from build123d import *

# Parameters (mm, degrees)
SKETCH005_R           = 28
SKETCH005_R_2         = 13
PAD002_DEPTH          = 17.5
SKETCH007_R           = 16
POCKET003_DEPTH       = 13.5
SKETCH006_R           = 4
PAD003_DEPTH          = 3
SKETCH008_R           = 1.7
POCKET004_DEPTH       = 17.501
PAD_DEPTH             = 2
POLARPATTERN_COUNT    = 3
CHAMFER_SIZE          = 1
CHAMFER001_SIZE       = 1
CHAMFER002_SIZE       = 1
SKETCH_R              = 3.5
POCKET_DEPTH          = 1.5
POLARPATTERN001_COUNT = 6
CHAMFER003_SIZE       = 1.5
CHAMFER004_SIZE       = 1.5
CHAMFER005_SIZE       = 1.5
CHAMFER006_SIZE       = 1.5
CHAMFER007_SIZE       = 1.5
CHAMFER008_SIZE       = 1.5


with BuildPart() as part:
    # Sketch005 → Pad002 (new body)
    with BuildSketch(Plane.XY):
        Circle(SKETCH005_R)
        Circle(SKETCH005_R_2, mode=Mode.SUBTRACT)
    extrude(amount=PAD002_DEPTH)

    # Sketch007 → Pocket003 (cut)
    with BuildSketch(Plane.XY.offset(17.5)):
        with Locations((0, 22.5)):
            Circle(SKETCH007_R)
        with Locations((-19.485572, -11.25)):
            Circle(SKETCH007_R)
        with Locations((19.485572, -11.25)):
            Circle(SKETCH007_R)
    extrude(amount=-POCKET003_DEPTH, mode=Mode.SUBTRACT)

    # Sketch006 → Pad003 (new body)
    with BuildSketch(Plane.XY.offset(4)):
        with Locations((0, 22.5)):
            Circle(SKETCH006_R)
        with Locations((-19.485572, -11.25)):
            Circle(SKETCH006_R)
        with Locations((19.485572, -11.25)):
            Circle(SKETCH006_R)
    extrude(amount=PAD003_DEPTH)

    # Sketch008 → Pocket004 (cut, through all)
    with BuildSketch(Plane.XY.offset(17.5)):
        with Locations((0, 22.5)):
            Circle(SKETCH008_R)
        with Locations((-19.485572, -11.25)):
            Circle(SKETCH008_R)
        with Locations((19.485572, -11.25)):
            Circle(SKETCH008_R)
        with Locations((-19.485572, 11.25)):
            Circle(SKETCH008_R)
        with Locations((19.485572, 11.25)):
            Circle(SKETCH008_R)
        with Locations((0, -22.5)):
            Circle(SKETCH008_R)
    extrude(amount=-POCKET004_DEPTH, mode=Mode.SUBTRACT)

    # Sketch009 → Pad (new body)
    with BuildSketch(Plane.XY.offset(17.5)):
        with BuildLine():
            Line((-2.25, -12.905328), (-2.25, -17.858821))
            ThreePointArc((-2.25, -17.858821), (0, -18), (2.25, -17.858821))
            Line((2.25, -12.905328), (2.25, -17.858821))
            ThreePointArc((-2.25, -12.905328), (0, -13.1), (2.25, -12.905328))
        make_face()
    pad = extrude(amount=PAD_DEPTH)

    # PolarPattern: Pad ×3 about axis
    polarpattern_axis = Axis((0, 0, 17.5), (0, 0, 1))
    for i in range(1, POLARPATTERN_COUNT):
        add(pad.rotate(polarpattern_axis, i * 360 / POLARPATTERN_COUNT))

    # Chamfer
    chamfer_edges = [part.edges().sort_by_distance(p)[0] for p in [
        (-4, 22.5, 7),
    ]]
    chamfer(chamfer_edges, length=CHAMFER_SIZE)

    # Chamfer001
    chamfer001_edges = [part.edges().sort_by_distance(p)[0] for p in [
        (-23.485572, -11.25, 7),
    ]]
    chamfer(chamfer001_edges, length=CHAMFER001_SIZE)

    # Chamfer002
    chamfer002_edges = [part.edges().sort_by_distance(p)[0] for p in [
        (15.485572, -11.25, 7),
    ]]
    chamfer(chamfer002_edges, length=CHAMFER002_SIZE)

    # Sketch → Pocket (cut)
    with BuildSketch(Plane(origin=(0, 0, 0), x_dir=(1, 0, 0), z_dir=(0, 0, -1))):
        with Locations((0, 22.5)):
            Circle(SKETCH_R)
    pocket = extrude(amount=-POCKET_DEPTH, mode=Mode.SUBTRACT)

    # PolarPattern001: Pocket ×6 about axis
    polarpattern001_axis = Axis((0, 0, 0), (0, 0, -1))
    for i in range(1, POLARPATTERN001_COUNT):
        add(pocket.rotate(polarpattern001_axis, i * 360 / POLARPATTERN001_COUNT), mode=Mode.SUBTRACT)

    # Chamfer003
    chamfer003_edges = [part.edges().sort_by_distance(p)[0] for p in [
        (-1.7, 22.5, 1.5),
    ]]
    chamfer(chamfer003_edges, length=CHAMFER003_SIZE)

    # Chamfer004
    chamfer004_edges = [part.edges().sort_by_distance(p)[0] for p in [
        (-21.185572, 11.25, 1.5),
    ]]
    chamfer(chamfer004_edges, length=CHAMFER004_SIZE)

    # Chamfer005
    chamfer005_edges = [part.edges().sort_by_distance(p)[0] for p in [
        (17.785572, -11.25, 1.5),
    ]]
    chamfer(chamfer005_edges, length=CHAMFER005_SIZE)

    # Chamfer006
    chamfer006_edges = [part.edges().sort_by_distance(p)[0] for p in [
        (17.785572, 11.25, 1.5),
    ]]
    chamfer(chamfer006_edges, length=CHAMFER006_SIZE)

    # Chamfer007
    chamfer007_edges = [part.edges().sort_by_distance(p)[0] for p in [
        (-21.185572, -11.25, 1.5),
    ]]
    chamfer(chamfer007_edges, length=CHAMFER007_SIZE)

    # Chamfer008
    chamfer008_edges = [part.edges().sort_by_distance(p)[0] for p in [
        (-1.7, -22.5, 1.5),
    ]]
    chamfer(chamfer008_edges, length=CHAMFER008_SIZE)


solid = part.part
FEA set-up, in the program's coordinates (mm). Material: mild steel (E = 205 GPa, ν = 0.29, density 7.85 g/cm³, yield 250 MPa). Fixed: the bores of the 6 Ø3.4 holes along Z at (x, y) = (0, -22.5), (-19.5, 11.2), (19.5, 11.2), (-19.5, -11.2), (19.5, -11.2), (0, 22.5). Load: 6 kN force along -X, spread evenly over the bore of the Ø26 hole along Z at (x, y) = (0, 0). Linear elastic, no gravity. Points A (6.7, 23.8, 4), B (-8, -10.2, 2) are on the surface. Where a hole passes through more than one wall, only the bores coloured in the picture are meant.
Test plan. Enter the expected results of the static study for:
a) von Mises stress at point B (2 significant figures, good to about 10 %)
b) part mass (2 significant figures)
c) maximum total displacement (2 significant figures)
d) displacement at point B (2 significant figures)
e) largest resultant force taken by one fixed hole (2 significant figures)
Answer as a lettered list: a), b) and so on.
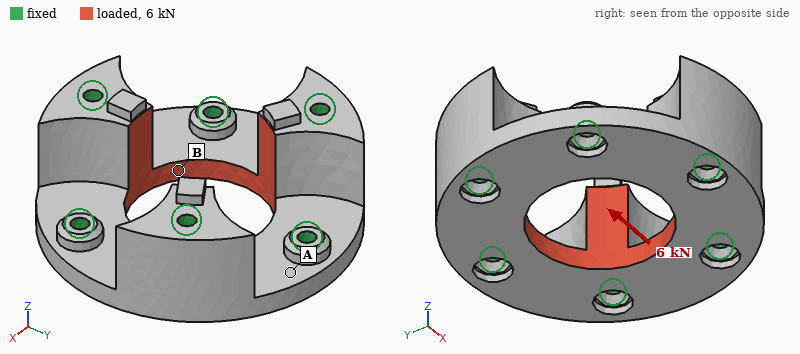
a) 16 MPa
b) 120 g
c) 2.9 µm
d) 1.4 µm
e) 1.6 kN
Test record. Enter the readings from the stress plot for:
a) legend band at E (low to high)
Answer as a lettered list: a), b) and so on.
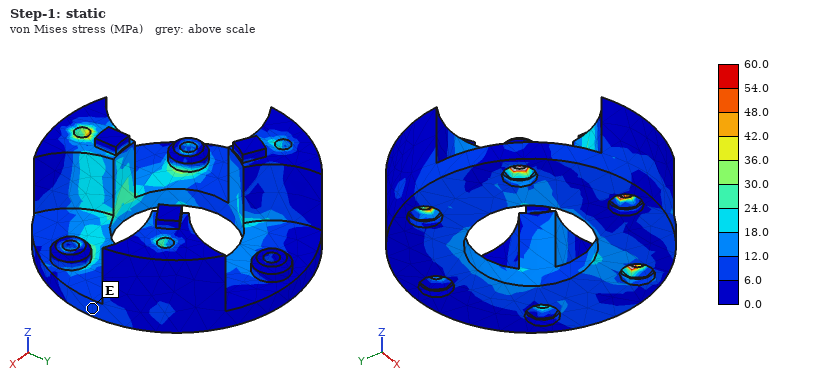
a) 6.0 to 12.0 MPa
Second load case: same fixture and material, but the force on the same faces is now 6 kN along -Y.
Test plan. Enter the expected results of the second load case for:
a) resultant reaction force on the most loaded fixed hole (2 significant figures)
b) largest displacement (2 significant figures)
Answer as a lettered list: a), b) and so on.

a) 1.6 kN
b) 2.6 µm
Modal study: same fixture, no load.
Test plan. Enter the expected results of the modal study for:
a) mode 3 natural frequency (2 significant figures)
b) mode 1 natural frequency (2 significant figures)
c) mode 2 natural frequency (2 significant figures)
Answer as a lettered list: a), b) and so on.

a) 41 kHz
b) 40 kHz
c) 40 kHz
